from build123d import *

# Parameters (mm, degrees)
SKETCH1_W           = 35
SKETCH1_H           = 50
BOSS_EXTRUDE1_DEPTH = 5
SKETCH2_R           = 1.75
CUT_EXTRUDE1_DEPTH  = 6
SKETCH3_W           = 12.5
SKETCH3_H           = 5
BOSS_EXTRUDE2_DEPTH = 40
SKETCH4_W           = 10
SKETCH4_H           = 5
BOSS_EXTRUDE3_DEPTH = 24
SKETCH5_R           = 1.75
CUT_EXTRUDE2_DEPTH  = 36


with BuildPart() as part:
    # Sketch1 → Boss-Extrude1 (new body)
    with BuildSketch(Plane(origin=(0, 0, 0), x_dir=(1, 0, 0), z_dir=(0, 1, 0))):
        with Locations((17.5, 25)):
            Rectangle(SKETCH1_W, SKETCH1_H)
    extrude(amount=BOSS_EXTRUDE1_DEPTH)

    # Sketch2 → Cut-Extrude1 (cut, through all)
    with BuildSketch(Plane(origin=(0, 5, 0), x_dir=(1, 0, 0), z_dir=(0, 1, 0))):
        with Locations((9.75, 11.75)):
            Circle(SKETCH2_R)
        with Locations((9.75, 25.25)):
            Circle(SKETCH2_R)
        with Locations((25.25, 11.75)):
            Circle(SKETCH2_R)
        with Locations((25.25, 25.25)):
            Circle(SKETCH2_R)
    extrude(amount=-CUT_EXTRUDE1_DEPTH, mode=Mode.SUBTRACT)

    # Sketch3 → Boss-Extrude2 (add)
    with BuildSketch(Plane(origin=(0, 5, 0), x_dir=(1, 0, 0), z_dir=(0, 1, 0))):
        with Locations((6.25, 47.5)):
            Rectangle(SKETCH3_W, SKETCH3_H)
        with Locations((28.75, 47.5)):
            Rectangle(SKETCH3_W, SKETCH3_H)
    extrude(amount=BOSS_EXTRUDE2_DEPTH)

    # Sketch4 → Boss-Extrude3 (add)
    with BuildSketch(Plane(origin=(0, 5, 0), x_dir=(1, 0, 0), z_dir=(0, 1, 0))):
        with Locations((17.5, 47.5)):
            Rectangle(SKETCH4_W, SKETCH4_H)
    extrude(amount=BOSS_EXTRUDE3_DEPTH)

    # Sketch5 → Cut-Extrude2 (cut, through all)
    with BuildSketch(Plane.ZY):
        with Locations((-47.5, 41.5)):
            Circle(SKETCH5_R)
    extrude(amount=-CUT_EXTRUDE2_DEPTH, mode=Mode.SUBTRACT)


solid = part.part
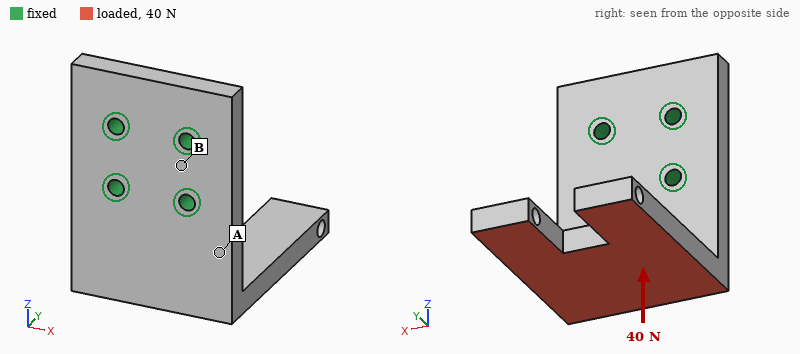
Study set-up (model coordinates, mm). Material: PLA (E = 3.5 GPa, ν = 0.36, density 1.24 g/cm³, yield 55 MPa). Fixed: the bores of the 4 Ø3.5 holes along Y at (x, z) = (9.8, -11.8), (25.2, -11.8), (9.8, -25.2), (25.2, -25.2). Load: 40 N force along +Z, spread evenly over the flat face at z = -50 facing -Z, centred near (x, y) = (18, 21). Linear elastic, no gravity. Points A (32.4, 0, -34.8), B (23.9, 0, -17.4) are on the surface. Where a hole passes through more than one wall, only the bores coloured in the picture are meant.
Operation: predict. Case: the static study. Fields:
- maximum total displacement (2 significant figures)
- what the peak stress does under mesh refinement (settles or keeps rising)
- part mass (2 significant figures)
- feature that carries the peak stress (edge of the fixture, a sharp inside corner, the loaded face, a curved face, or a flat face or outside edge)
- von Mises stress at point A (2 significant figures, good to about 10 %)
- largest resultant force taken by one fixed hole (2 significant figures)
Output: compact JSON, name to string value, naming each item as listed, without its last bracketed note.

{"maximum total displacement": "0.73 mm", "what the peak stress does under mesh refinement": "keeps rising", "part mass": "18 g", "feature that carries the peak stress": "edge of the fixture", "von Mises stress at point A": "4.7 MPa", "largest resultant force taken by one fixed hole": "19 N"}
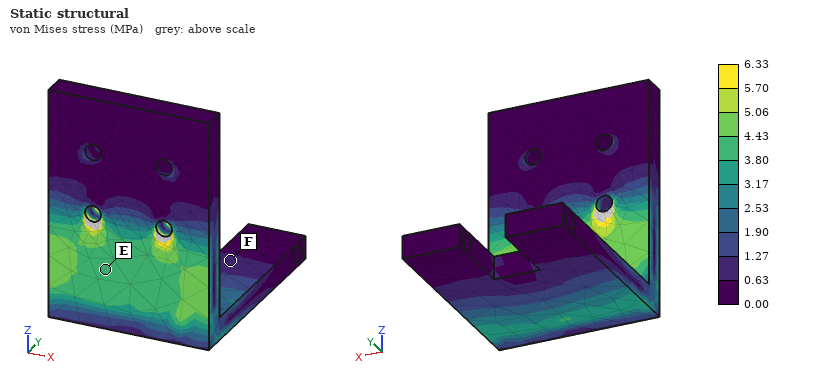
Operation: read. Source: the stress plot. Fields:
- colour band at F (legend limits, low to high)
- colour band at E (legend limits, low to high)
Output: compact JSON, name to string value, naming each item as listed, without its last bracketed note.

{"colour band at F": "0.63 to 1.27 MPa", "colour band at E": "3.80 to 4.43 MPa"}
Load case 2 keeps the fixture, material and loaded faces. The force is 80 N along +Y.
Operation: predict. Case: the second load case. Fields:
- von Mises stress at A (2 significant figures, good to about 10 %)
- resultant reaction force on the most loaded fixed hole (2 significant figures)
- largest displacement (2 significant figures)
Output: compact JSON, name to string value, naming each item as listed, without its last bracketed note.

{"von Mises stress at A": "7.9 MPa", "resultant reaction force on the most loaded fixed hole": "62 N", "largest displacement": "0.91 mm"}
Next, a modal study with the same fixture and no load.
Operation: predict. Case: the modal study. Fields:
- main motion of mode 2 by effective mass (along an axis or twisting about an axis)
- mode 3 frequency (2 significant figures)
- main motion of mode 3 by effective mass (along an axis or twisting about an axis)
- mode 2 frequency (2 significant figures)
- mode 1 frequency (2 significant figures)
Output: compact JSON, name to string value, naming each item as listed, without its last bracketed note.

{"main motion of mode 2 by effective mass": "along X", "mode 3 frequency": "1500 Hz", "main motion of mode 3 by effective mass": "along Y", "mode 2 frequency": "840 Hz", "mode 1 frequency": "500 Hz"}
